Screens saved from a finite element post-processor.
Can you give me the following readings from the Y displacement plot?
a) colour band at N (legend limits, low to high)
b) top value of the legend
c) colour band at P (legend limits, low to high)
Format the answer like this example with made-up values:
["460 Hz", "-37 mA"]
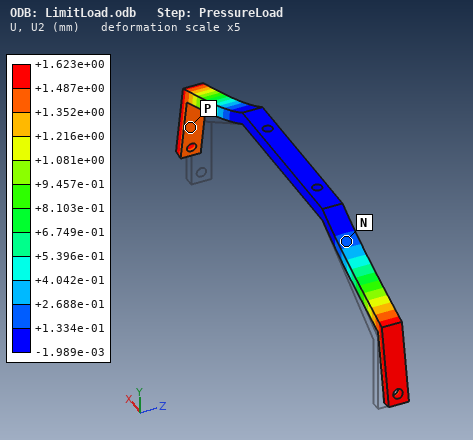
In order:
["+1.334e-01 to +2.688e-01 mm", "+1.623e+00 mm", "+1.352e+00 to +1.487e+00 mm"]
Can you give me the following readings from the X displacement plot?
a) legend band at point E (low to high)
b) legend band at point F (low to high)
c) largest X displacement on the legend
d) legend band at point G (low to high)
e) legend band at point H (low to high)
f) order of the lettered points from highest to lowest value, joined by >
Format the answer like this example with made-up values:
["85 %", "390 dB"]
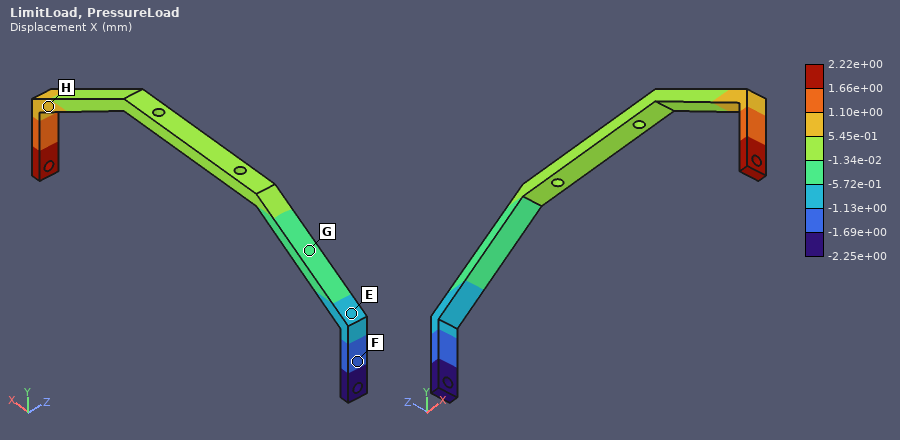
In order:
["-1.13e+00 to -5.72e-01 mm", "-1.69e+00 to -1.13e+00 mm", "2.22e+00 mm", "-5.72e-01 to -1.34e-02 mm", "5.45e-01 to 1.10e+00 mm", "H > G > E > F"]
